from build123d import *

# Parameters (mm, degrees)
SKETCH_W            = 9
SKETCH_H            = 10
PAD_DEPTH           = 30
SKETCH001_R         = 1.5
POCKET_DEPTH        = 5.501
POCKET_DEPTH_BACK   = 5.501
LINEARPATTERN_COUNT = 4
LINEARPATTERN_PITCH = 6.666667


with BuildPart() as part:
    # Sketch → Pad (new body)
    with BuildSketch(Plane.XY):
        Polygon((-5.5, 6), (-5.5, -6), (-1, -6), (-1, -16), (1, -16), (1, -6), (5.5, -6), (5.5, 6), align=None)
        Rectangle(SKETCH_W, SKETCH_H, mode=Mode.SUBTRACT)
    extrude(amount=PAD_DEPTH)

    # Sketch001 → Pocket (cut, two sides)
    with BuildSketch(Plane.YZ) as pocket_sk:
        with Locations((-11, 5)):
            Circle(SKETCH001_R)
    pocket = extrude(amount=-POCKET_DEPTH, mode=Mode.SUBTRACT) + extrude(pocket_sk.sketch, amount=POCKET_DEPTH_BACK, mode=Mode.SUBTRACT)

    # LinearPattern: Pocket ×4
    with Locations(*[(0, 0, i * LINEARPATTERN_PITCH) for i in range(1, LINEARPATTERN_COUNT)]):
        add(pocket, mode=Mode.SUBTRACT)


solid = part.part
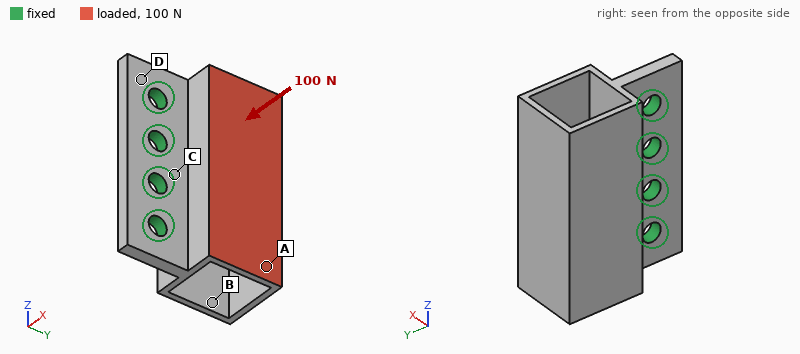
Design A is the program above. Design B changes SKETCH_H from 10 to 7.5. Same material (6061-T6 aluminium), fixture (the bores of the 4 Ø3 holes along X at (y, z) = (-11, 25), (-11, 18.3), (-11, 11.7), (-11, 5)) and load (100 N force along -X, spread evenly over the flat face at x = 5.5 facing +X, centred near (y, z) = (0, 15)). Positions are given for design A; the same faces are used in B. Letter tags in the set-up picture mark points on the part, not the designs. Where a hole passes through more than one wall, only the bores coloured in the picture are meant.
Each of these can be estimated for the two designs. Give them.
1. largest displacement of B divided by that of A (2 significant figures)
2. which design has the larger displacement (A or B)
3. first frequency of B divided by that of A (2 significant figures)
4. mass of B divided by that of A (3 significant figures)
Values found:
0.50
A
1.2
1.37
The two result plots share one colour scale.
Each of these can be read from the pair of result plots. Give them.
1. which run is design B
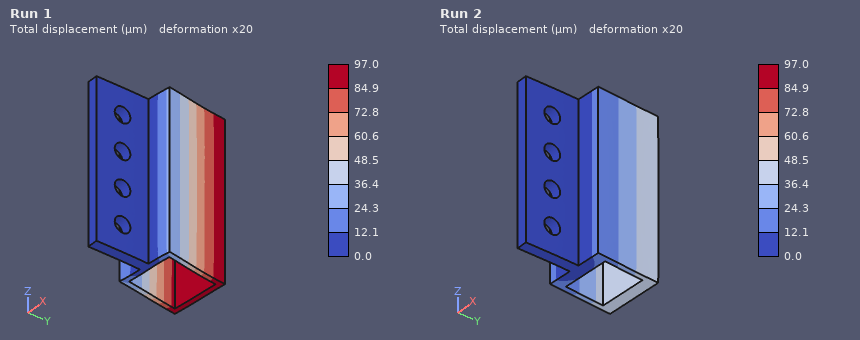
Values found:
Run 2
